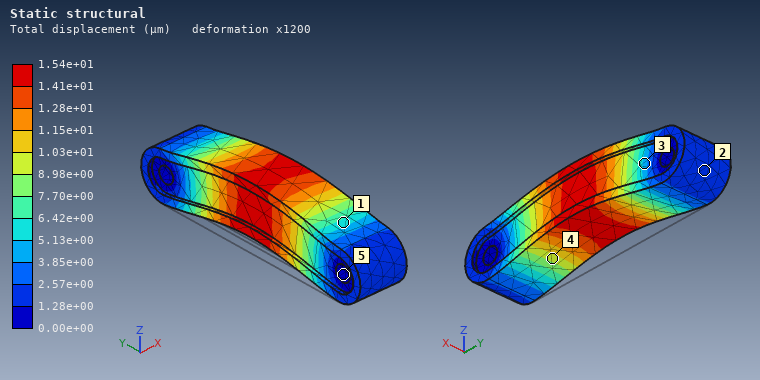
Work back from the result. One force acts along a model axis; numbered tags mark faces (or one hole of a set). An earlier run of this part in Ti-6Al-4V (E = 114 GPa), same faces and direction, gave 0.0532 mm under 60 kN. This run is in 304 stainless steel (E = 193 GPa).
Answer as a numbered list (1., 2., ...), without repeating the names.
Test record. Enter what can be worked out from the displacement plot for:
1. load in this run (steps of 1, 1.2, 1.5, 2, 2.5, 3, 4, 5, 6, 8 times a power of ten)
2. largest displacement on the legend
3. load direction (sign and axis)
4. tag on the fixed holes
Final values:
1. 30 kN
2. 1.54e+01 µm
3. +Z
4. 5
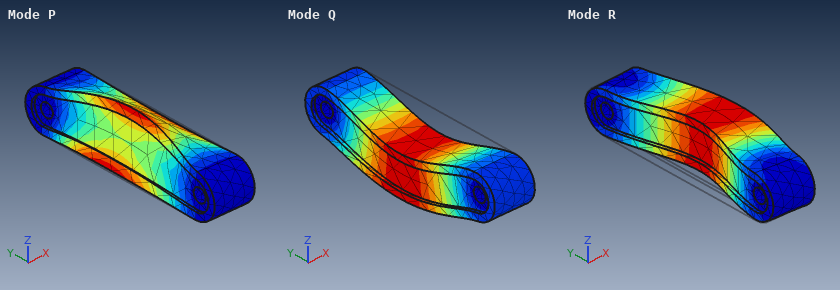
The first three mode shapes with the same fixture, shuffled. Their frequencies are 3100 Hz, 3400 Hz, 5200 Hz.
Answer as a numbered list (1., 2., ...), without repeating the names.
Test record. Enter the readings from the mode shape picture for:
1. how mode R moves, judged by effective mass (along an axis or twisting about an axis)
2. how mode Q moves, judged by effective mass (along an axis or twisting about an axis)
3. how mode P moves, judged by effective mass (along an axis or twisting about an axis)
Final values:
1. along X
2. along Z
3. twisting about Y
